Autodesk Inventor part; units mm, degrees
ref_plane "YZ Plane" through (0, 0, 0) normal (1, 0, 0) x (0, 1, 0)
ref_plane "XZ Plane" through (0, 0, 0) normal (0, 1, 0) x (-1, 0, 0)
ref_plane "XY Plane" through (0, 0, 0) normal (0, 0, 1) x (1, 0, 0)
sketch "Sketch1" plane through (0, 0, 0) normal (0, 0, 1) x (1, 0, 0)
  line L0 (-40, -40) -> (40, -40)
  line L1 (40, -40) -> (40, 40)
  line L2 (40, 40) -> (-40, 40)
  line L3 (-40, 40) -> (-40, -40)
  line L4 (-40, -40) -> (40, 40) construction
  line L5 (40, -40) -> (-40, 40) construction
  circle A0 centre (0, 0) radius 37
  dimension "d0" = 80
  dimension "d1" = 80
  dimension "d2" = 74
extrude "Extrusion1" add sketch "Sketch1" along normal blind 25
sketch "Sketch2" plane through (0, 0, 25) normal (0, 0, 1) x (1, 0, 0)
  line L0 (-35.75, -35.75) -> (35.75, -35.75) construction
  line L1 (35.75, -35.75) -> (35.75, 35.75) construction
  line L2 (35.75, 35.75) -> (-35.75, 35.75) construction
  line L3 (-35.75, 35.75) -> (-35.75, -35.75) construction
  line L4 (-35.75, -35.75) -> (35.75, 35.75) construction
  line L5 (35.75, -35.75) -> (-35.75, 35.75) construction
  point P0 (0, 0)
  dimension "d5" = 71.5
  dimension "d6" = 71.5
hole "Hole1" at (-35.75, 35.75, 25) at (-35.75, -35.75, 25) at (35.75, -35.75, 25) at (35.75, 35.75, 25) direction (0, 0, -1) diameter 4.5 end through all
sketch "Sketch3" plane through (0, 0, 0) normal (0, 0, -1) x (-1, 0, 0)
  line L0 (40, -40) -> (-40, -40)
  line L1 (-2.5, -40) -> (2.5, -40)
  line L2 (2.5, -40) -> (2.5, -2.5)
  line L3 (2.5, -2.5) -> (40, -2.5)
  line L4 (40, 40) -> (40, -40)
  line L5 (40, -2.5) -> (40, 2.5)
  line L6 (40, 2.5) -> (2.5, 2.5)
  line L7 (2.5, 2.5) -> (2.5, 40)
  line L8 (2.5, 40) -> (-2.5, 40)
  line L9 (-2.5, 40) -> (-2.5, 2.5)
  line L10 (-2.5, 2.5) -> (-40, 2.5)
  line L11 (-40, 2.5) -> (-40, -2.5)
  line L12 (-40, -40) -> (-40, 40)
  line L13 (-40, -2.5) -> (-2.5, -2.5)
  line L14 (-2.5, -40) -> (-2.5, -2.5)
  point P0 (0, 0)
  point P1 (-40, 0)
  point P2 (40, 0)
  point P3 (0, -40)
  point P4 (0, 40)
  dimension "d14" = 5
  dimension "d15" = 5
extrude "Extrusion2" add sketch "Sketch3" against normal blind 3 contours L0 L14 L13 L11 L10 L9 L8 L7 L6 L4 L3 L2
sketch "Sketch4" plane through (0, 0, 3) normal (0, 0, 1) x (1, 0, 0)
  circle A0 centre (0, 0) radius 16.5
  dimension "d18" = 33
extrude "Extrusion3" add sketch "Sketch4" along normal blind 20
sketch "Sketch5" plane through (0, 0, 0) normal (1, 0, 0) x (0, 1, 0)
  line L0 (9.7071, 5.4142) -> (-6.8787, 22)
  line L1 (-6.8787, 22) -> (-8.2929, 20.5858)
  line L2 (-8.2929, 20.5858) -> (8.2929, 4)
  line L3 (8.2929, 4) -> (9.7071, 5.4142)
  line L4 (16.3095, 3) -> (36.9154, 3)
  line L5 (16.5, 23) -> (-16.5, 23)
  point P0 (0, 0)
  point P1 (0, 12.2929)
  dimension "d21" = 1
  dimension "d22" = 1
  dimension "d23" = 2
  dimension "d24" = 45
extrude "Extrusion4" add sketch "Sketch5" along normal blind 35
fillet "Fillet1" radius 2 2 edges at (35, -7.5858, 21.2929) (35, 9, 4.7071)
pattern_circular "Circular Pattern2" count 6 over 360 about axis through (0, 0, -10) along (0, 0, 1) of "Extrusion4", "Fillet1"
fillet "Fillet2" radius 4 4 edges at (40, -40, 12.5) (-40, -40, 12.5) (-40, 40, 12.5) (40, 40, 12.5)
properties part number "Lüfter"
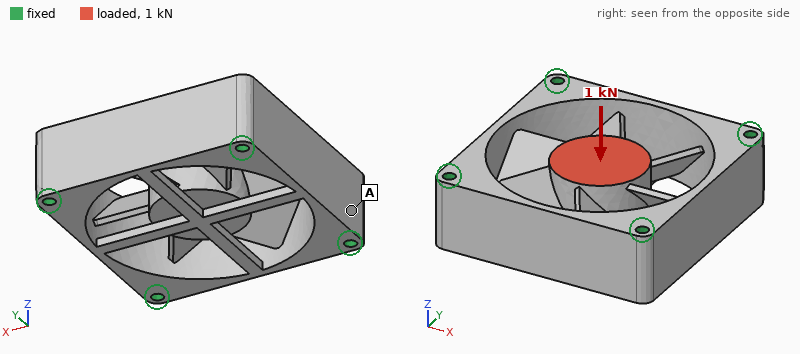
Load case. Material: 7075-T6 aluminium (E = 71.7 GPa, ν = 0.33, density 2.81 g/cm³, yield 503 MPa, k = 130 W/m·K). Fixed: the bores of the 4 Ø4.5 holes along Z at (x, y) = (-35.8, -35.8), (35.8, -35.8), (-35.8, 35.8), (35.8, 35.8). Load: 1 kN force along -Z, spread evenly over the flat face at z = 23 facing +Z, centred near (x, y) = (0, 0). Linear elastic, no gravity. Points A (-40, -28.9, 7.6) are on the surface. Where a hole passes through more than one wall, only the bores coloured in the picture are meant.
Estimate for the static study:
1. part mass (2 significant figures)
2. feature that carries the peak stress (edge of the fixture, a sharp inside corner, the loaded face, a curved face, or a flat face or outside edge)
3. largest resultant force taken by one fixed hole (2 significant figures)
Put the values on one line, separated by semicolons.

210 g; a flat face or outside edge; 250 N
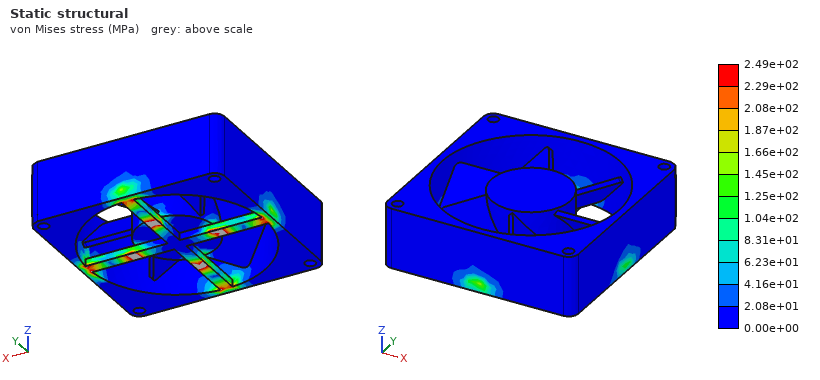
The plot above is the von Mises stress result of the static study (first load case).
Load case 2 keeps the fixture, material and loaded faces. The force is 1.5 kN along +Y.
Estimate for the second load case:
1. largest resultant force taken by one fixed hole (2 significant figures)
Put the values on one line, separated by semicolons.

700 N
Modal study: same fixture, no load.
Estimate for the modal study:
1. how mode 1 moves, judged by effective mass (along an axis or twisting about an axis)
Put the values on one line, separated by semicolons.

along Z
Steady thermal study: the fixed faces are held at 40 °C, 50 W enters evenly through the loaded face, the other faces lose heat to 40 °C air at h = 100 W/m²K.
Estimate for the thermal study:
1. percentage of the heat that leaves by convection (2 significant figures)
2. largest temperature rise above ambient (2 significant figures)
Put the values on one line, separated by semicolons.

81 %; 48 K
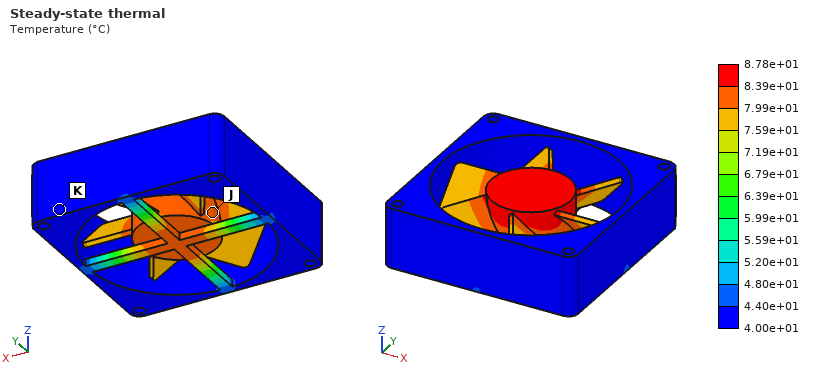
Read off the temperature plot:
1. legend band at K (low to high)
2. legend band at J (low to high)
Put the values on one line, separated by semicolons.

4.00e+01 to 4.40e+01 °C; 7.99e+01 to 8.39e+01 °C
